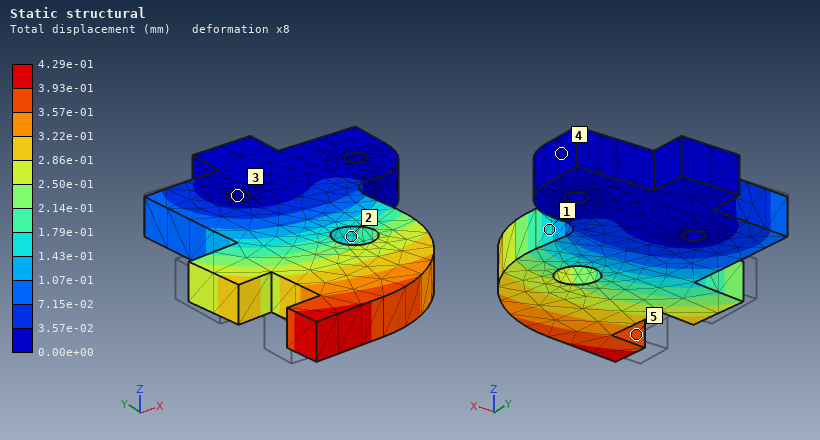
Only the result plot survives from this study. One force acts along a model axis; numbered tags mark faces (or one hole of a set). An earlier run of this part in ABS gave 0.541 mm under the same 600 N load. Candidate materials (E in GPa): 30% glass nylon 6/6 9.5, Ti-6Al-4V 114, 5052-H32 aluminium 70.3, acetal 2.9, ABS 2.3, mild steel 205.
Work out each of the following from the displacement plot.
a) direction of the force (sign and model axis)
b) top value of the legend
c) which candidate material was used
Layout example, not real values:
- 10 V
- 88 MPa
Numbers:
- +X
- 4.29e-01 mm
- acetal
